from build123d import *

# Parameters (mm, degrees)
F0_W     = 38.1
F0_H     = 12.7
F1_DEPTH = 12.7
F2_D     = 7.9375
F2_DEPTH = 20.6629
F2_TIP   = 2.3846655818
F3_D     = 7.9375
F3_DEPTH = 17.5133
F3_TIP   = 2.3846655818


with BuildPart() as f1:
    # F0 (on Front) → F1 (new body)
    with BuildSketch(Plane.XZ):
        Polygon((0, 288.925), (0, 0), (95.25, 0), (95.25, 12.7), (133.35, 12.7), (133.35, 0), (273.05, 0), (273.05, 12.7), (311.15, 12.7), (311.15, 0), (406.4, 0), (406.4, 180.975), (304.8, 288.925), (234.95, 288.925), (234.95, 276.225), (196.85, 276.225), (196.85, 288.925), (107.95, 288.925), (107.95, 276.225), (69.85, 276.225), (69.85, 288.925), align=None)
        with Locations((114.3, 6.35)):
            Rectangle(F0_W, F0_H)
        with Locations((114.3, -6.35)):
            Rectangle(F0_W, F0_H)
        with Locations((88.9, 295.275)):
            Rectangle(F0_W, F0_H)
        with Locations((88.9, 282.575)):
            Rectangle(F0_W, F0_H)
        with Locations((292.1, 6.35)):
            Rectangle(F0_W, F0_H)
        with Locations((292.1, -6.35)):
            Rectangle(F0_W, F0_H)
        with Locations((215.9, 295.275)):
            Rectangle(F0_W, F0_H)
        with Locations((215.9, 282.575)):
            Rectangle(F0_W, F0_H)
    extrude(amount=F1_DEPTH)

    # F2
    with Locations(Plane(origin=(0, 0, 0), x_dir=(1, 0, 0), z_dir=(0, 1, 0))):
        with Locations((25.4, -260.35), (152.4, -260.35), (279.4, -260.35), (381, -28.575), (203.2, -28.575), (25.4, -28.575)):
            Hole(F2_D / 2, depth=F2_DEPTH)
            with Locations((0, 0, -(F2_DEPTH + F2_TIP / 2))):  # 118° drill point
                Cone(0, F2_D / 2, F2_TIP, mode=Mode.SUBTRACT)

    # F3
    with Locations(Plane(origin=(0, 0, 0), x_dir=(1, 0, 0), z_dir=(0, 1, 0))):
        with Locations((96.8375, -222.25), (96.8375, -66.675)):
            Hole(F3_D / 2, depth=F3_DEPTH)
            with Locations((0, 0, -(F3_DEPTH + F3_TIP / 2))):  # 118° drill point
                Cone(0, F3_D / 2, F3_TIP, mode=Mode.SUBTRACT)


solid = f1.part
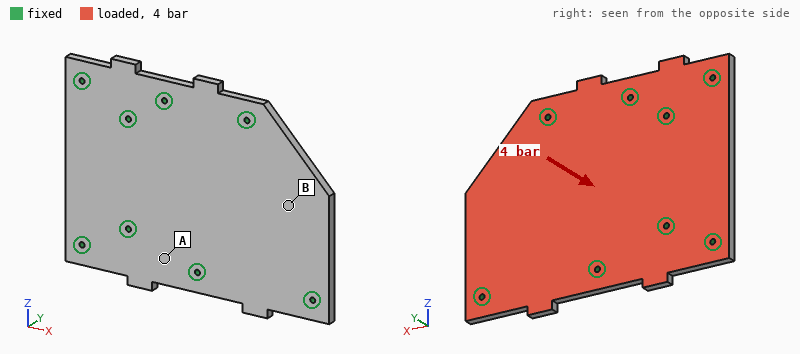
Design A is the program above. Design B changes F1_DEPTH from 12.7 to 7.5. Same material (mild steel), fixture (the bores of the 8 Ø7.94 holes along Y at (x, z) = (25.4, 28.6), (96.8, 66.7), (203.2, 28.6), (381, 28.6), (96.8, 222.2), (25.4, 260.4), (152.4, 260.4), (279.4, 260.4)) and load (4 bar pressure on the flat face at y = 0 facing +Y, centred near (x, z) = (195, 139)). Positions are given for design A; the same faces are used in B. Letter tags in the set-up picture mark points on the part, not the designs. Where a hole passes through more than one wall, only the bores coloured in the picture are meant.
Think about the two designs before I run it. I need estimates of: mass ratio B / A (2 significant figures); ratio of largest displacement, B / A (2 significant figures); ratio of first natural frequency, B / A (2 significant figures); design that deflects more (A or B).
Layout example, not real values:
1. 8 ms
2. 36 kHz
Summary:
1. 0.59
2. 4.5
3. 0.62
4. B
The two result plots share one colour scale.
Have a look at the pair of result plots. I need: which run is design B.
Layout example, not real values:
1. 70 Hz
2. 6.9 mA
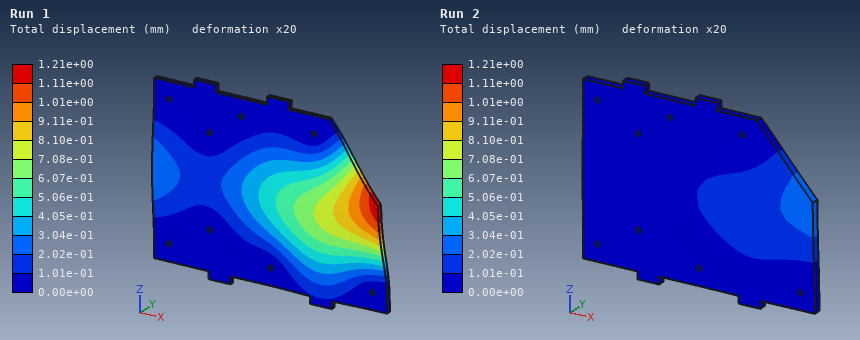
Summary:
1. Run 1
